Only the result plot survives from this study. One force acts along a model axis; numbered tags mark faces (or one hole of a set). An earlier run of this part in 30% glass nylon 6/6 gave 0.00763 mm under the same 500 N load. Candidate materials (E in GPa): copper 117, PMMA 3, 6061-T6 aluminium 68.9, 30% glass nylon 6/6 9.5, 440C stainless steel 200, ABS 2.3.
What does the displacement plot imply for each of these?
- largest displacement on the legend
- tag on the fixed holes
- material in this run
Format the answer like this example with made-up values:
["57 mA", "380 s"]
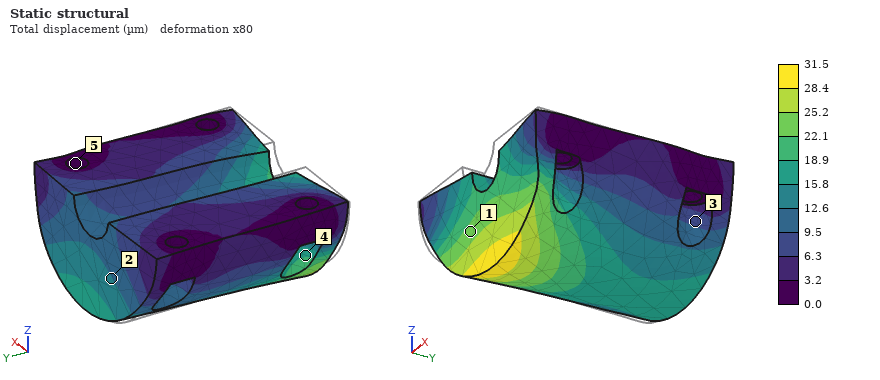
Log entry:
["31.5 µm", "5", "ABS"]
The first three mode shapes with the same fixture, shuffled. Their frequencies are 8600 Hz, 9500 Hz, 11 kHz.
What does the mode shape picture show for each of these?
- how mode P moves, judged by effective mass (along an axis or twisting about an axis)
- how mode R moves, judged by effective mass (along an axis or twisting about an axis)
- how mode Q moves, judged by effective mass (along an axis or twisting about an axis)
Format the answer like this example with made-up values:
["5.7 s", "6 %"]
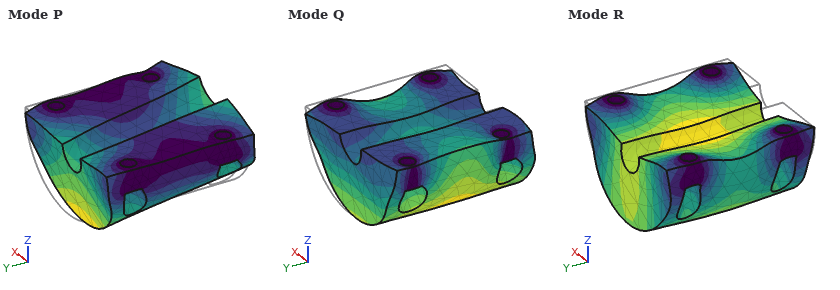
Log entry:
["along Y", "along Z", "along X"]
